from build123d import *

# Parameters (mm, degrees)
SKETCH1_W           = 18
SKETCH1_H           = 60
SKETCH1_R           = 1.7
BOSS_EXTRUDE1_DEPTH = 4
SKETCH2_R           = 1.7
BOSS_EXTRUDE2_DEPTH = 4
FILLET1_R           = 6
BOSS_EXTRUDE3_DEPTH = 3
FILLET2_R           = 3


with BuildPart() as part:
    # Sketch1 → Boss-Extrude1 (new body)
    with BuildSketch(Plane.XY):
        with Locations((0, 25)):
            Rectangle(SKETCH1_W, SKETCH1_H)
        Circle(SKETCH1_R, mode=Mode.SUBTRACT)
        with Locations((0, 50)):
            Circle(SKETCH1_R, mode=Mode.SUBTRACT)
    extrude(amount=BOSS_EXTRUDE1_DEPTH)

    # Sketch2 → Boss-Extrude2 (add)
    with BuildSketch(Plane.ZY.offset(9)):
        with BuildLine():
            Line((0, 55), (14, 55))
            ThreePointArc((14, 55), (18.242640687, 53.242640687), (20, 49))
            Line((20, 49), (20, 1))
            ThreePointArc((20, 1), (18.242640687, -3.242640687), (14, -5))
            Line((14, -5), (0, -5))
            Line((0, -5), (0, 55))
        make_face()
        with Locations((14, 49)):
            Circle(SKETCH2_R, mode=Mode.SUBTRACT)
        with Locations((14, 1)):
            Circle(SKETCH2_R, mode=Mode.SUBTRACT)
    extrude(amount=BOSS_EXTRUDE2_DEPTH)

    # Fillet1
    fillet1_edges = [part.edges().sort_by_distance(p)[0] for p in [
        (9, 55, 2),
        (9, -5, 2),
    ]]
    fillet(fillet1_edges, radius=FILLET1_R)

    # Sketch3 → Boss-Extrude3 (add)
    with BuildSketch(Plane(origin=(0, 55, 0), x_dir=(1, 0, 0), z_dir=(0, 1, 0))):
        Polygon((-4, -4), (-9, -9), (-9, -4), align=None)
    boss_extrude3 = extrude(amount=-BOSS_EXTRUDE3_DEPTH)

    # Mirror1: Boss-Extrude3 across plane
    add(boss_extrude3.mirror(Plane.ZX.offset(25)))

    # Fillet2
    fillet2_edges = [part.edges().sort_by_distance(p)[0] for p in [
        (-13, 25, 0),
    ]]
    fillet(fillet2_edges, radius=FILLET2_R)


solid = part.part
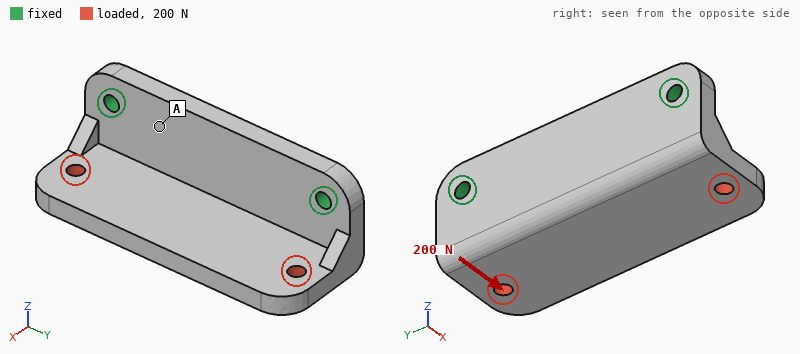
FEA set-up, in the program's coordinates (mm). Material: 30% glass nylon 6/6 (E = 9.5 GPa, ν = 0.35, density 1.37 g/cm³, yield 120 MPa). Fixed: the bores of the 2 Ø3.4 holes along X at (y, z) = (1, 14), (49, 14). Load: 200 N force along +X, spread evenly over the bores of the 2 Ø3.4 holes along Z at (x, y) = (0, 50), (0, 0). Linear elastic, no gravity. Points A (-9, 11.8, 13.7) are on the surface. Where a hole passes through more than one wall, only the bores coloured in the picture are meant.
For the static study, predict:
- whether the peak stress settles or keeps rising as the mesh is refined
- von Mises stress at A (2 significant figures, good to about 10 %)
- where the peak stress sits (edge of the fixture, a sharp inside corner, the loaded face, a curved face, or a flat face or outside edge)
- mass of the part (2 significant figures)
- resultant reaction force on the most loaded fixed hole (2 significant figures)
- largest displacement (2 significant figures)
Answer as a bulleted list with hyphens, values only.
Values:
- keeps rising
- 5.2 MPa
- edge of the fixture
- 12 g
- 100 N
- 0.17 mm
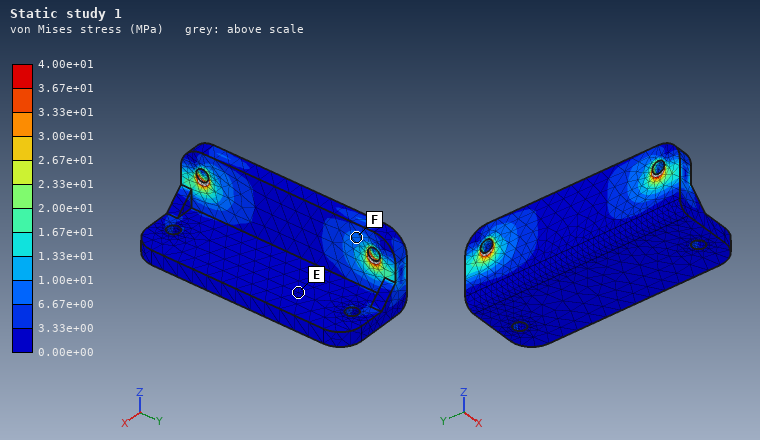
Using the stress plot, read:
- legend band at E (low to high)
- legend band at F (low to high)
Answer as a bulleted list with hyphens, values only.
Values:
- 0.00e+00 to 3.33e+00 MPa
- 6.67e+00 to 1.00e+01 MPa
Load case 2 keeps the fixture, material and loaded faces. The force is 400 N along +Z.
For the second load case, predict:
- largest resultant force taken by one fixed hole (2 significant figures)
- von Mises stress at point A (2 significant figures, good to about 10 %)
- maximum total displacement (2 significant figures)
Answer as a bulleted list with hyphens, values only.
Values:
- 200 N
- 15 MPa
- 0.57 mm
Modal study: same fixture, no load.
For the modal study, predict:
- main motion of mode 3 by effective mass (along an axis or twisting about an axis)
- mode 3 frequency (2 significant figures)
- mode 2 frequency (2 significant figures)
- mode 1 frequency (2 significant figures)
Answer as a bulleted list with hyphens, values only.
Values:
- along X
- 4700 Hz
- 3400 Hz
- 1900 Hz
